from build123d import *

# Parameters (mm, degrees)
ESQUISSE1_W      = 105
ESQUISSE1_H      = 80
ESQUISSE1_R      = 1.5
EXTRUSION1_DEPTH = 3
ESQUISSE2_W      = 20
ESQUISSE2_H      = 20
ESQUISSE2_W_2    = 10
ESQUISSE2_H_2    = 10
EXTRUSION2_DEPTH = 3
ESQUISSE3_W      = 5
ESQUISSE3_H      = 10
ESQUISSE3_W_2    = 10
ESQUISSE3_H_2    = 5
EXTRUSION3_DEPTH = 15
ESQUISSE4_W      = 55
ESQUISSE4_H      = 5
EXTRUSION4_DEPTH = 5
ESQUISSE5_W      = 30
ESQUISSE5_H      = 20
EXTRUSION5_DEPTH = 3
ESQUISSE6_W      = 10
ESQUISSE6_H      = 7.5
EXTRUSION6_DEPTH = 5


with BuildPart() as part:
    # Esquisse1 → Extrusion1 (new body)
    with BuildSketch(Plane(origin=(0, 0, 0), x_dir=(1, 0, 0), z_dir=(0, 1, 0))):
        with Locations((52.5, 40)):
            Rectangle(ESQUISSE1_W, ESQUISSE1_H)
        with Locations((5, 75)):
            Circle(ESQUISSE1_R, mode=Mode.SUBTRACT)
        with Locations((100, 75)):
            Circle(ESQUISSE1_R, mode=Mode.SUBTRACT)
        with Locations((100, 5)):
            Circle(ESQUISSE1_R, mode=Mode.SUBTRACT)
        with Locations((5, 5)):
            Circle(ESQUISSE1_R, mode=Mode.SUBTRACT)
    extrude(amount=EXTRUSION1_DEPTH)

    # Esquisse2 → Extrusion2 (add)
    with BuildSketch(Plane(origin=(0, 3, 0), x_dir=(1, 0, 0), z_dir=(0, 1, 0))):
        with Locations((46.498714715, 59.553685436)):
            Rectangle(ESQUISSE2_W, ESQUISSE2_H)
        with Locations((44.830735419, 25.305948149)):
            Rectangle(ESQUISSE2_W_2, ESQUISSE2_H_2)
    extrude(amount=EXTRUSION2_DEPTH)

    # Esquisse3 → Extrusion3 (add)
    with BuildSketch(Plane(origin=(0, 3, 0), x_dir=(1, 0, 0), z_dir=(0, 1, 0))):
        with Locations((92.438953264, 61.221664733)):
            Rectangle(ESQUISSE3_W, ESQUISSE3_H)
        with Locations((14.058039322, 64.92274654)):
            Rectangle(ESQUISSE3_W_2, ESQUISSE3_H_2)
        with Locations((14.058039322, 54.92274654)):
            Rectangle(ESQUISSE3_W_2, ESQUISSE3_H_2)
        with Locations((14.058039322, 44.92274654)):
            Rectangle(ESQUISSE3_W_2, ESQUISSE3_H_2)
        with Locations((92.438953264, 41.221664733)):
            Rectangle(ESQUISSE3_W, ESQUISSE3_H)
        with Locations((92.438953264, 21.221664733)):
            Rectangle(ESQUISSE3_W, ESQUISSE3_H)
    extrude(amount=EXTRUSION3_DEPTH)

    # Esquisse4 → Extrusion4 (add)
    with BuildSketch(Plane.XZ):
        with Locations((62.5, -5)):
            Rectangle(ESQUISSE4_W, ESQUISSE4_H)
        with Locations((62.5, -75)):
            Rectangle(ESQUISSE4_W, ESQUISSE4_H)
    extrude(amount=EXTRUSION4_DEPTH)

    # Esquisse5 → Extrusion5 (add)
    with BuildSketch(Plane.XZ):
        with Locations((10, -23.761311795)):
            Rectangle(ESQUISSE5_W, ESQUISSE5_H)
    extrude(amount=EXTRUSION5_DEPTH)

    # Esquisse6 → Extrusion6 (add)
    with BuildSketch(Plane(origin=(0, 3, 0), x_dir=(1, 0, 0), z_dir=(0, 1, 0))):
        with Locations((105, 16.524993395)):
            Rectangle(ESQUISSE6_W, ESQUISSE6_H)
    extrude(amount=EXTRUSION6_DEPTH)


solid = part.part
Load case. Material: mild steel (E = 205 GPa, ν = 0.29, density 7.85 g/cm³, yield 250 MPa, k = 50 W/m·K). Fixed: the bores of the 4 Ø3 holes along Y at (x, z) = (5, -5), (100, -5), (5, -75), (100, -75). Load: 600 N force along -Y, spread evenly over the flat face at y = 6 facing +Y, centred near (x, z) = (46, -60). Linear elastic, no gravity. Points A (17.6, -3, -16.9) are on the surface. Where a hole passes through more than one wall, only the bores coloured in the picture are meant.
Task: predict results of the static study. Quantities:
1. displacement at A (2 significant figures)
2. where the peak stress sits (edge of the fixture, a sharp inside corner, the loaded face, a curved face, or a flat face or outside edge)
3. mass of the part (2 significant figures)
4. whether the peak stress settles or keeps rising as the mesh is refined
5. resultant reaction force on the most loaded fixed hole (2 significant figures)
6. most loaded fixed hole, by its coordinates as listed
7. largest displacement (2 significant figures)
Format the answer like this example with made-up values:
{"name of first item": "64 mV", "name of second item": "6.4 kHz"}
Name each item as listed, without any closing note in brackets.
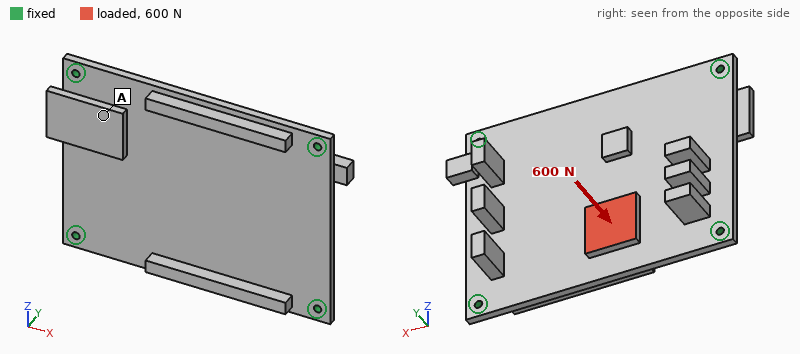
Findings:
{"displacement at A": "20 µm", "where the peak stress sits": "edge of the fixture", "mass of the part": "280 g", "whether the peak stress settles or keeps rising as the mesh is refined": "keeps rising", "resultant reaction force on the most loaded fixed hole": "320 N", "most loaded fixed hole, by its coordinates as listed": "(5, -75)", "largest displacement": "70 µm"}
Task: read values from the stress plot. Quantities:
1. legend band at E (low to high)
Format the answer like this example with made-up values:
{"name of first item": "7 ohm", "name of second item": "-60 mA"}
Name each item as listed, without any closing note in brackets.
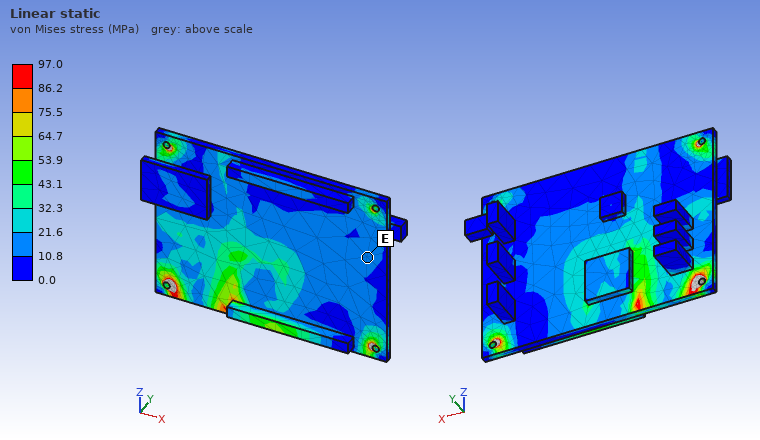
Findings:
{"legend band at E": "10.8 to 21.6 MPa"}
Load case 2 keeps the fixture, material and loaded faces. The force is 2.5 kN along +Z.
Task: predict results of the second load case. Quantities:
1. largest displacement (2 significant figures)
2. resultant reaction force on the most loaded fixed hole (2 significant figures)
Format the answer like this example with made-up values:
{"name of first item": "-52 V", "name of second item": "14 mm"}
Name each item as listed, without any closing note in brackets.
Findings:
{"largest displacement": "42 µm", "resultant reaction force on the most loaded fixed hole": "800 N"}
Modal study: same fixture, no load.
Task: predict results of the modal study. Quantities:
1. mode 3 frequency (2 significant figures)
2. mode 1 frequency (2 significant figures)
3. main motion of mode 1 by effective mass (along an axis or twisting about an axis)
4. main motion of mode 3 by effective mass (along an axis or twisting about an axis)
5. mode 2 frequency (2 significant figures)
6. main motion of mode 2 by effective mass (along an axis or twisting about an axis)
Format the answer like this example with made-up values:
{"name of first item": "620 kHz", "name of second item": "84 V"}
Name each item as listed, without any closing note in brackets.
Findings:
{"mode 3 frequency": "2700 Hz", "mode 1 frequency": "1400 Hz", "main motion of mode 1 by effective mass": "along Y", "main motion of mode 3 by effective mass": "twisting about Z", "mode 2 frequency": "2500 Hz", "main motion of mode 2 by effective mass": "twisting about X"}
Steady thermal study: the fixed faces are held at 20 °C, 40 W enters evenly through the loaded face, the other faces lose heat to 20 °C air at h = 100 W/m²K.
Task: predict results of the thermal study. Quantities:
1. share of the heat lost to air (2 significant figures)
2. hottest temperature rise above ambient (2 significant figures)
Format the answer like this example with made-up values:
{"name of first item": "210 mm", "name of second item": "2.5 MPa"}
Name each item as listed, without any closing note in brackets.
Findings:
{"share of the heat lost to air": "82 %", "hottest temperature rise above ambient": "70 K"}
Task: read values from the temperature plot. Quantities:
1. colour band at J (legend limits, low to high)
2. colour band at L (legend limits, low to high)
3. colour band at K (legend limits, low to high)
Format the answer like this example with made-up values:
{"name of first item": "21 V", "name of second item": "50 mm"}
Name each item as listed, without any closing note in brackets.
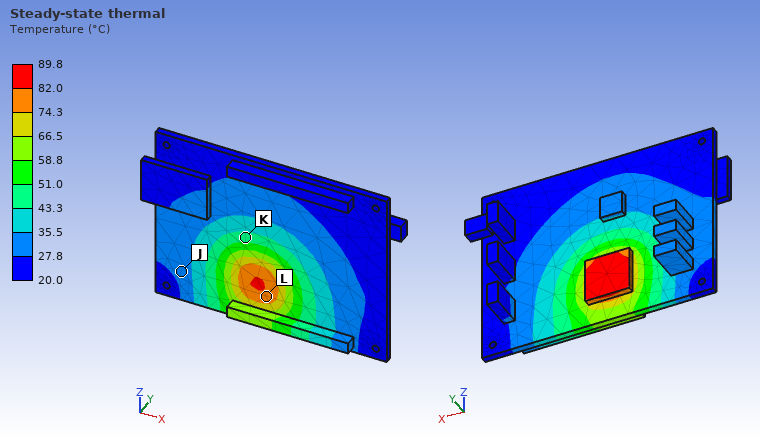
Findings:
{"colour band at J": "27.8 to 35.5 °C", "colour band at L": "74.3 to 82.0 °C", "colour band at K": "43.3 to 51.0 °C"}
